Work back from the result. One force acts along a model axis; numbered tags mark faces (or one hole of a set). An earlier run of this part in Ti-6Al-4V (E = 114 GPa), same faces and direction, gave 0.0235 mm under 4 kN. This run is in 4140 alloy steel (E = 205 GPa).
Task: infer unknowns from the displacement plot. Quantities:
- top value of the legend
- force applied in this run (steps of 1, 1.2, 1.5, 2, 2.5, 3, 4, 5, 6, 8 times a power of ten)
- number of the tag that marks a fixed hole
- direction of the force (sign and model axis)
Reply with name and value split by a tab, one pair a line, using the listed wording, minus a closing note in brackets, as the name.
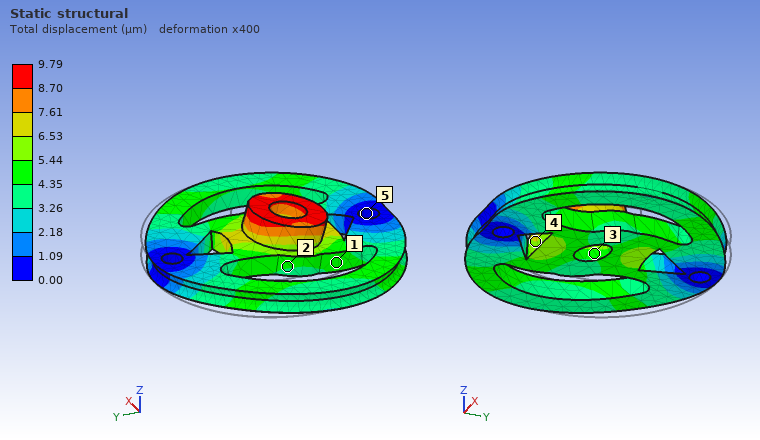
top value of the legend	9.79 µm
force applied in this run	3 kN
number of the tag that marks a fixed hole	5
direction of the force	-Y
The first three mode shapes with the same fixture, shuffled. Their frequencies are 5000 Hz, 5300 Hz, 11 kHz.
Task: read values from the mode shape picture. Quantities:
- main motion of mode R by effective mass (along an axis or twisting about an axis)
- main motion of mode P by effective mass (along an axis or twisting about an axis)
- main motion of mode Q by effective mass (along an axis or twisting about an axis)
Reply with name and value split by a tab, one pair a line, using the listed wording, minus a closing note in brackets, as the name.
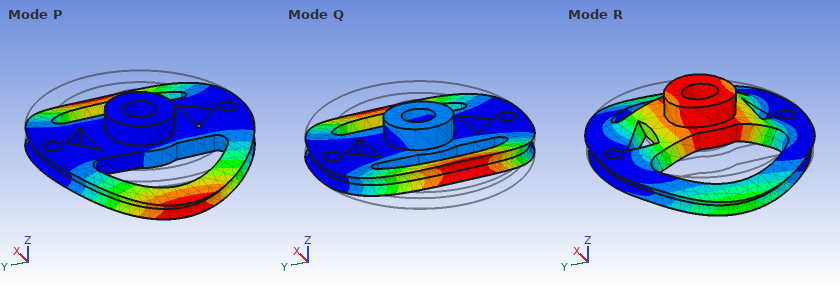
main motion of mode R by effective mass	along Z
main motion of mode P by effective mass	along Z
main motion of mode Q by effective mass	twisting about Y
